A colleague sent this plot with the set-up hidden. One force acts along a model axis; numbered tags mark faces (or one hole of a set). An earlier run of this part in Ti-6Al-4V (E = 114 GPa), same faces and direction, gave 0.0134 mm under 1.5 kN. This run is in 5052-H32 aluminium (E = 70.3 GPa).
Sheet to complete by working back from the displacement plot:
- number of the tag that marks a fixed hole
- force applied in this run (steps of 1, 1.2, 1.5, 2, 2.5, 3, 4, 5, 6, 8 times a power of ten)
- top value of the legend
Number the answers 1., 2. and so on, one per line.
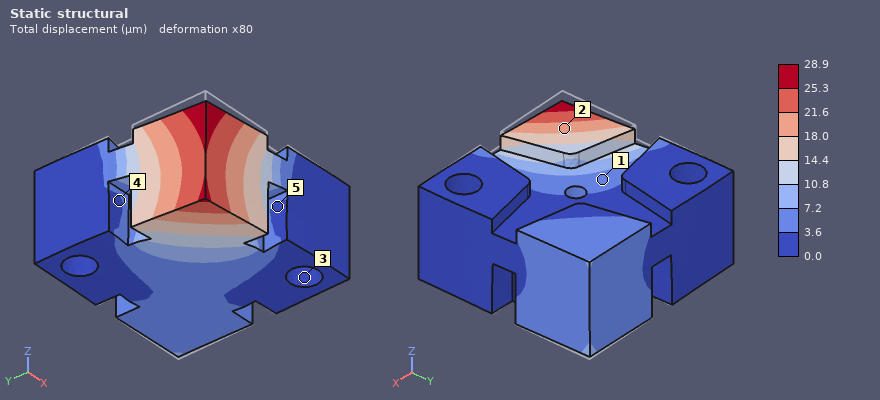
1. 3
2. 2 kN
3. 28.9 µm
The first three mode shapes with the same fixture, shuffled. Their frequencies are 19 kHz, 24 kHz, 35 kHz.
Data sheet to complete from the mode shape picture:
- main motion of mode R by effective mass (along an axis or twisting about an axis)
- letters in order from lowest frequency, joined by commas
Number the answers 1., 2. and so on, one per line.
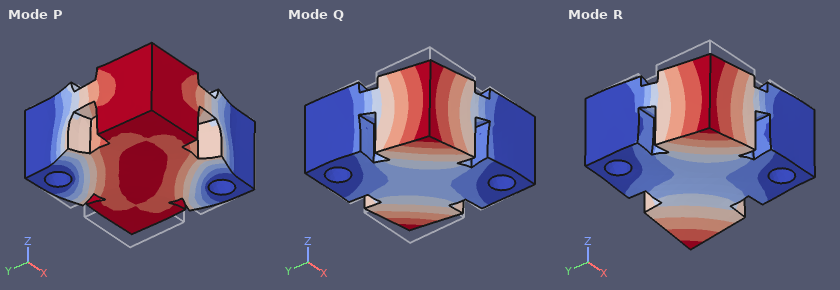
1. along Z
2. Q, R, P
